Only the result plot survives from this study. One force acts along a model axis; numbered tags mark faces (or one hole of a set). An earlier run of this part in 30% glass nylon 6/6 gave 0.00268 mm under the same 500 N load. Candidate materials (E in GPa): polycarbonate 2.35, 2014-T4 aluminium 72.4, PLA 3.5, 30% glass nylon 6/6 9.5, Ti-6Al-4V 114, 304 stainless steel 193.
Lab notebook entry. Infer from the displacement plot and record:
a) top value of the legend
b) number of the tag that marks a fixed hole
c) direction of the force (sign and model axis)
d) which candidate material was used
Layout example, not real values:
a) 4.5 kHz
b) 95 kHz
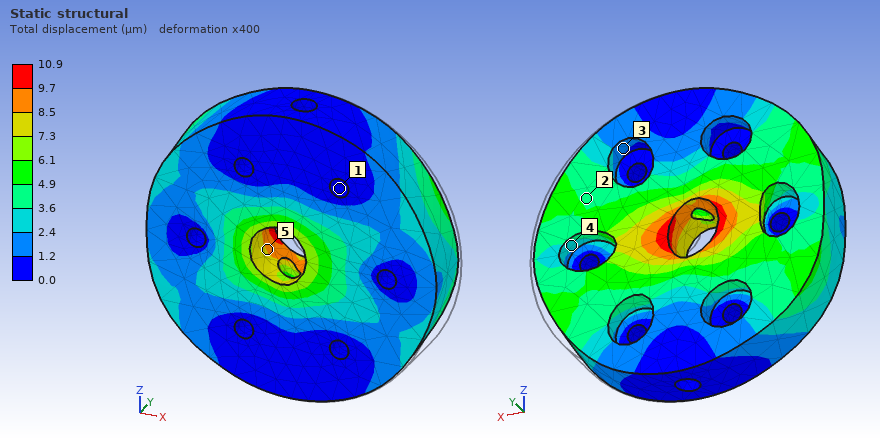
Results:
a) 10.9 µm
b) 1
c) -X
d) polycarbonate
